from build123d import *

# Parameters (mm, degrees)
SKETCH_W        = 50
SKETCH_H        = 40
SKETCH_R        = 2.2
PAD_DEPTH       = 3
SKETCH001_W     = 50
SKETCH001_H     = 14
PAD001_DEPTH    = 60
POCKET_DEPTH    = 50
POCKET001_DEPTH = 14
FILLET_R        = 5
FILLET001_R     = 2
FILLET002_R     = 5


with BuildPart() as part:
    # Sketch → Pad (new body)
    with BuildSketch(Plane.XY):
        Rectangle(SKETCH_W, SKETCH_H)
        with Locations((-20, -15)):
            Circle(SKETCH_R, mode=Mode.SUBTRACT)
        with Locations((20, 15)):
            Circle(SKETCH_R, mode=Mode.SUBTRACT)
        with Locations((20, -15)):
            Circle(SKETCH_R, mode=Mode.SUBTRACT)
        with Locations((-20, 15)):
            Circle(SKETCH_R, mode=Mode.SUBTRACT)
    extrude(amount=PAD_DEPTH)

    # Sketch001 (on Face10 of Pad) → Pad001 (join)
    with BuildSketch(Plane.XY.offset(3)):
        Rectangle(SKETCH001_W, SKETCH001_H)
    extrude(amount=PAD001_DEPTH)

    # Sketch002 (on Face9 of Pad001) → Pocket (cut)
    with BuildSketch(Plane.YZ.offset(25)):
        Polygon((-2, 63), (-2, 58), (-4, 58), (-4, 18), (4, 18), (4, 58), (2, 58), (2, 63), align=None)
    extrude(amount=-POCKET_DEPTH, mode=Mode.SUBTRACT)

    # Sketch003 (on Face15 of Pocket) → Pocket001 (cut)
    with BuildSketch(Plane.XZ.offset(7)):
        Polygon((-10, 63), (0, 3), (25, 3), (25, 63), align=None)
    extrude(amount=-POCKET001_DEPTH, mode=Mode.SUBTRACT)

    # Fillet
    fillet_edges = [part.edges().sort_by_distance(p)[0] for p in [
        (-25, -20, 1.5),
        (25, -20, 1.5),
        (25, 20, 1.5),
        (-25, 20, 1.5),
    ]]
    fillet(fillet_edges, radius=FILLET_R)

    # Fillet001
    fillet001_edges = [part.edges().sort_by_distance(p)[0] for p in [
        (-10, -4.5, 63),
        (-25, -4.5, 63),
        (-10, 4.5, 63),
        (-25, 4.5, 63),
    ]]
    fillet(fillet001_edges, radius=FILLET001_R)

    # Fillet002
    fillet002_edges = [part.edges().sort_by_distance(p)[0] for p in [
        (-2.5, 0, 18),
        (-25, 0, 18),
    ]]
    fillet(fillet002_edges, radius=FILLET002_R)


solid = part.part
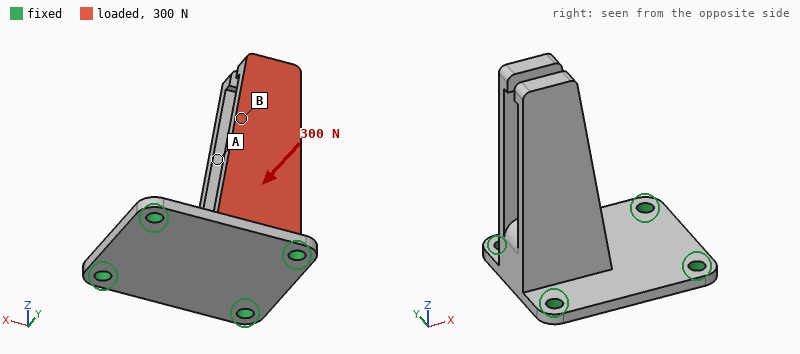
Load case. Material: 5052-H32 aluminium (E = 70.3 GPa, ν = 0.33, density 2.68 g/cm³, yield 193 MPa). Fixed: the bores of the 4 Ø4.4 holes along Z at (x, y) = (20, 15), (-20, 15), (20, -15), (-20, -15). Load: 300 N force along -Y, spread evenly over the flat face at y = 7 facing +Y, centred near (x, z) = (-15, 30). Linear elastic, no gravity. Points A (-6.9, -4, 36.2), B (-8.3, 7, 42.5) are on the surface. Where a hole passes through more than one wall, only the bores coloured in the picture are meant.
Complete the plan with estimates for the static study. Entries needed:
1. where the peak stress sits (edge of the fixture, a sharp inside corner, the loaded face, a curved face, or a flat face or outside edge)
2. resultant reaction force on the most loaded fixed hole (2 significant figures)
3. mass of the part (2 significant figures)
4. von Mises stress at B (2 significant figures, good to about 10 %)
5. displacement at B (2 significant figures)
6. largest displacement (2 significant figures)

the loaded face
370 N
43 g
34 MPa
0.35 mm
0.82 mm
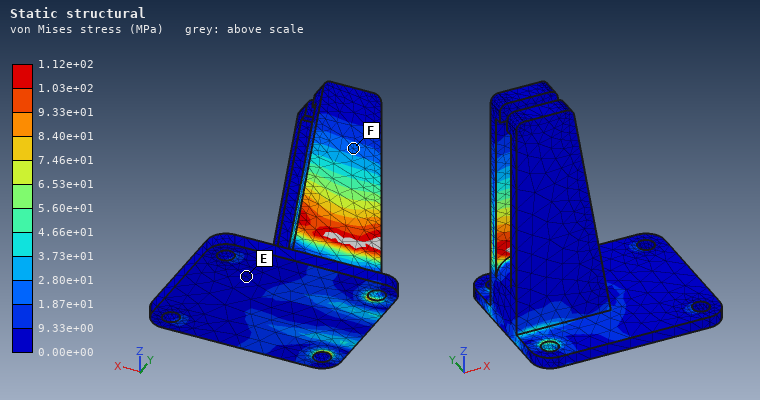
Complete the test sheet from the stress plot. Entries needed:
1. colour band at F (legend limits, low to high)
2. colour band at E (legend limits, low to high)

1.87e+01 to 2.80e+01 MPa
0.00e+00 to 9.33e+00 MPa
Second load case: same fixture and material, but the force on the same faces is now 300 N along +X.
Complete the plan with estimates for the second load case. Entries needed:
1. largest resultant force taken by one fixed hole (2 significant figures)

160 N
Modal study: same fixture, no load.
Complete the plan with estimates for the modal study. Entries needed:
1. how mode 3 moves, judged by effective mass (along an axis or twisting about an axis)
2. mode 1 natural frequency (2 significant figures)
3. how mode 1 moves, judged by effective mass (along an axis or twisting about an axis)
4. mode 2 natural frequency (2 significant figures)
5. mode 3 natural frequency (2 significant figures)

along X
1100 Hz
along Y
1200 Hz
2100 Hz
